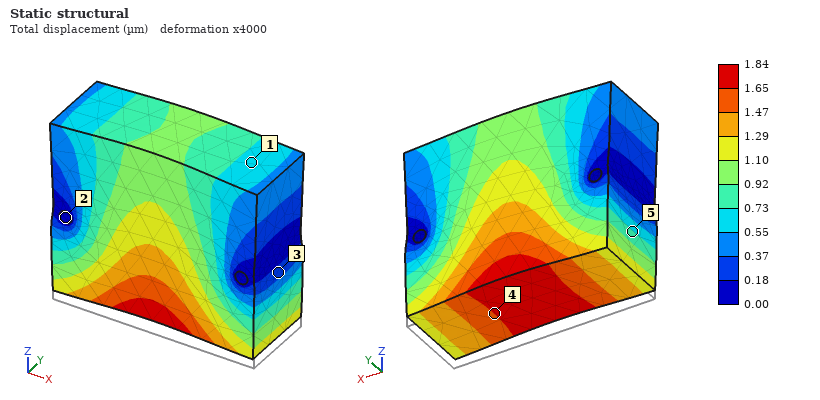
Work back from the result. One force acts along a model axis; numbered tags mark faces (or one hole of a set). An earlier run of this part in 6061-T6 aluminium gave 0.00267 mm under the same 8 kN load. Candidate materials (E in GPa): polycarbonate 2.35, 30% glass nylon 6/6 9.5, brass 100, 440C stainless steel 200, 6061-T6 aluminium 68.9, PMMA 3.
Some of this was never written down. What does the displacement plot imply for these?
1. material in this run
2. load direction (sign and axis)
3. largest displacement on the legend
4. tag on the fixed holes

brass
+Z
1.84 µm
2
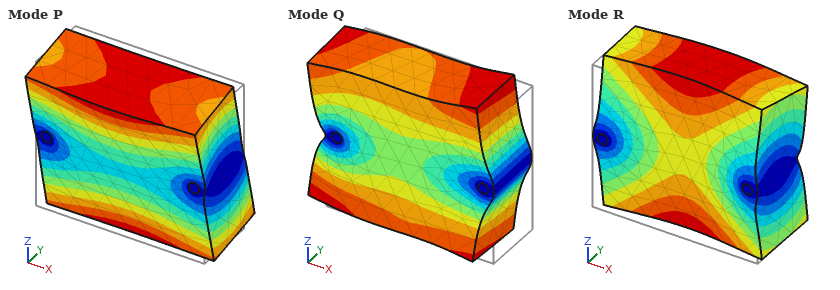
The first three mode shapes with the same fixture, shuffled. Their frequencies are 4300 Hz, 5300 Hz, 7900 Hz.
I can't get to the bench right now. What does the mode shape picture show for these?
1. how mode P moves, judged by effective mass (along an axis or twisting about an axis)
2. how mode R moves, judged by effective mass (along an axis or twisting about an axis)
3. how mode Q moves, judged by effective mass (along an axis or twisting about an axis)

twisting about X
along Y
along X
